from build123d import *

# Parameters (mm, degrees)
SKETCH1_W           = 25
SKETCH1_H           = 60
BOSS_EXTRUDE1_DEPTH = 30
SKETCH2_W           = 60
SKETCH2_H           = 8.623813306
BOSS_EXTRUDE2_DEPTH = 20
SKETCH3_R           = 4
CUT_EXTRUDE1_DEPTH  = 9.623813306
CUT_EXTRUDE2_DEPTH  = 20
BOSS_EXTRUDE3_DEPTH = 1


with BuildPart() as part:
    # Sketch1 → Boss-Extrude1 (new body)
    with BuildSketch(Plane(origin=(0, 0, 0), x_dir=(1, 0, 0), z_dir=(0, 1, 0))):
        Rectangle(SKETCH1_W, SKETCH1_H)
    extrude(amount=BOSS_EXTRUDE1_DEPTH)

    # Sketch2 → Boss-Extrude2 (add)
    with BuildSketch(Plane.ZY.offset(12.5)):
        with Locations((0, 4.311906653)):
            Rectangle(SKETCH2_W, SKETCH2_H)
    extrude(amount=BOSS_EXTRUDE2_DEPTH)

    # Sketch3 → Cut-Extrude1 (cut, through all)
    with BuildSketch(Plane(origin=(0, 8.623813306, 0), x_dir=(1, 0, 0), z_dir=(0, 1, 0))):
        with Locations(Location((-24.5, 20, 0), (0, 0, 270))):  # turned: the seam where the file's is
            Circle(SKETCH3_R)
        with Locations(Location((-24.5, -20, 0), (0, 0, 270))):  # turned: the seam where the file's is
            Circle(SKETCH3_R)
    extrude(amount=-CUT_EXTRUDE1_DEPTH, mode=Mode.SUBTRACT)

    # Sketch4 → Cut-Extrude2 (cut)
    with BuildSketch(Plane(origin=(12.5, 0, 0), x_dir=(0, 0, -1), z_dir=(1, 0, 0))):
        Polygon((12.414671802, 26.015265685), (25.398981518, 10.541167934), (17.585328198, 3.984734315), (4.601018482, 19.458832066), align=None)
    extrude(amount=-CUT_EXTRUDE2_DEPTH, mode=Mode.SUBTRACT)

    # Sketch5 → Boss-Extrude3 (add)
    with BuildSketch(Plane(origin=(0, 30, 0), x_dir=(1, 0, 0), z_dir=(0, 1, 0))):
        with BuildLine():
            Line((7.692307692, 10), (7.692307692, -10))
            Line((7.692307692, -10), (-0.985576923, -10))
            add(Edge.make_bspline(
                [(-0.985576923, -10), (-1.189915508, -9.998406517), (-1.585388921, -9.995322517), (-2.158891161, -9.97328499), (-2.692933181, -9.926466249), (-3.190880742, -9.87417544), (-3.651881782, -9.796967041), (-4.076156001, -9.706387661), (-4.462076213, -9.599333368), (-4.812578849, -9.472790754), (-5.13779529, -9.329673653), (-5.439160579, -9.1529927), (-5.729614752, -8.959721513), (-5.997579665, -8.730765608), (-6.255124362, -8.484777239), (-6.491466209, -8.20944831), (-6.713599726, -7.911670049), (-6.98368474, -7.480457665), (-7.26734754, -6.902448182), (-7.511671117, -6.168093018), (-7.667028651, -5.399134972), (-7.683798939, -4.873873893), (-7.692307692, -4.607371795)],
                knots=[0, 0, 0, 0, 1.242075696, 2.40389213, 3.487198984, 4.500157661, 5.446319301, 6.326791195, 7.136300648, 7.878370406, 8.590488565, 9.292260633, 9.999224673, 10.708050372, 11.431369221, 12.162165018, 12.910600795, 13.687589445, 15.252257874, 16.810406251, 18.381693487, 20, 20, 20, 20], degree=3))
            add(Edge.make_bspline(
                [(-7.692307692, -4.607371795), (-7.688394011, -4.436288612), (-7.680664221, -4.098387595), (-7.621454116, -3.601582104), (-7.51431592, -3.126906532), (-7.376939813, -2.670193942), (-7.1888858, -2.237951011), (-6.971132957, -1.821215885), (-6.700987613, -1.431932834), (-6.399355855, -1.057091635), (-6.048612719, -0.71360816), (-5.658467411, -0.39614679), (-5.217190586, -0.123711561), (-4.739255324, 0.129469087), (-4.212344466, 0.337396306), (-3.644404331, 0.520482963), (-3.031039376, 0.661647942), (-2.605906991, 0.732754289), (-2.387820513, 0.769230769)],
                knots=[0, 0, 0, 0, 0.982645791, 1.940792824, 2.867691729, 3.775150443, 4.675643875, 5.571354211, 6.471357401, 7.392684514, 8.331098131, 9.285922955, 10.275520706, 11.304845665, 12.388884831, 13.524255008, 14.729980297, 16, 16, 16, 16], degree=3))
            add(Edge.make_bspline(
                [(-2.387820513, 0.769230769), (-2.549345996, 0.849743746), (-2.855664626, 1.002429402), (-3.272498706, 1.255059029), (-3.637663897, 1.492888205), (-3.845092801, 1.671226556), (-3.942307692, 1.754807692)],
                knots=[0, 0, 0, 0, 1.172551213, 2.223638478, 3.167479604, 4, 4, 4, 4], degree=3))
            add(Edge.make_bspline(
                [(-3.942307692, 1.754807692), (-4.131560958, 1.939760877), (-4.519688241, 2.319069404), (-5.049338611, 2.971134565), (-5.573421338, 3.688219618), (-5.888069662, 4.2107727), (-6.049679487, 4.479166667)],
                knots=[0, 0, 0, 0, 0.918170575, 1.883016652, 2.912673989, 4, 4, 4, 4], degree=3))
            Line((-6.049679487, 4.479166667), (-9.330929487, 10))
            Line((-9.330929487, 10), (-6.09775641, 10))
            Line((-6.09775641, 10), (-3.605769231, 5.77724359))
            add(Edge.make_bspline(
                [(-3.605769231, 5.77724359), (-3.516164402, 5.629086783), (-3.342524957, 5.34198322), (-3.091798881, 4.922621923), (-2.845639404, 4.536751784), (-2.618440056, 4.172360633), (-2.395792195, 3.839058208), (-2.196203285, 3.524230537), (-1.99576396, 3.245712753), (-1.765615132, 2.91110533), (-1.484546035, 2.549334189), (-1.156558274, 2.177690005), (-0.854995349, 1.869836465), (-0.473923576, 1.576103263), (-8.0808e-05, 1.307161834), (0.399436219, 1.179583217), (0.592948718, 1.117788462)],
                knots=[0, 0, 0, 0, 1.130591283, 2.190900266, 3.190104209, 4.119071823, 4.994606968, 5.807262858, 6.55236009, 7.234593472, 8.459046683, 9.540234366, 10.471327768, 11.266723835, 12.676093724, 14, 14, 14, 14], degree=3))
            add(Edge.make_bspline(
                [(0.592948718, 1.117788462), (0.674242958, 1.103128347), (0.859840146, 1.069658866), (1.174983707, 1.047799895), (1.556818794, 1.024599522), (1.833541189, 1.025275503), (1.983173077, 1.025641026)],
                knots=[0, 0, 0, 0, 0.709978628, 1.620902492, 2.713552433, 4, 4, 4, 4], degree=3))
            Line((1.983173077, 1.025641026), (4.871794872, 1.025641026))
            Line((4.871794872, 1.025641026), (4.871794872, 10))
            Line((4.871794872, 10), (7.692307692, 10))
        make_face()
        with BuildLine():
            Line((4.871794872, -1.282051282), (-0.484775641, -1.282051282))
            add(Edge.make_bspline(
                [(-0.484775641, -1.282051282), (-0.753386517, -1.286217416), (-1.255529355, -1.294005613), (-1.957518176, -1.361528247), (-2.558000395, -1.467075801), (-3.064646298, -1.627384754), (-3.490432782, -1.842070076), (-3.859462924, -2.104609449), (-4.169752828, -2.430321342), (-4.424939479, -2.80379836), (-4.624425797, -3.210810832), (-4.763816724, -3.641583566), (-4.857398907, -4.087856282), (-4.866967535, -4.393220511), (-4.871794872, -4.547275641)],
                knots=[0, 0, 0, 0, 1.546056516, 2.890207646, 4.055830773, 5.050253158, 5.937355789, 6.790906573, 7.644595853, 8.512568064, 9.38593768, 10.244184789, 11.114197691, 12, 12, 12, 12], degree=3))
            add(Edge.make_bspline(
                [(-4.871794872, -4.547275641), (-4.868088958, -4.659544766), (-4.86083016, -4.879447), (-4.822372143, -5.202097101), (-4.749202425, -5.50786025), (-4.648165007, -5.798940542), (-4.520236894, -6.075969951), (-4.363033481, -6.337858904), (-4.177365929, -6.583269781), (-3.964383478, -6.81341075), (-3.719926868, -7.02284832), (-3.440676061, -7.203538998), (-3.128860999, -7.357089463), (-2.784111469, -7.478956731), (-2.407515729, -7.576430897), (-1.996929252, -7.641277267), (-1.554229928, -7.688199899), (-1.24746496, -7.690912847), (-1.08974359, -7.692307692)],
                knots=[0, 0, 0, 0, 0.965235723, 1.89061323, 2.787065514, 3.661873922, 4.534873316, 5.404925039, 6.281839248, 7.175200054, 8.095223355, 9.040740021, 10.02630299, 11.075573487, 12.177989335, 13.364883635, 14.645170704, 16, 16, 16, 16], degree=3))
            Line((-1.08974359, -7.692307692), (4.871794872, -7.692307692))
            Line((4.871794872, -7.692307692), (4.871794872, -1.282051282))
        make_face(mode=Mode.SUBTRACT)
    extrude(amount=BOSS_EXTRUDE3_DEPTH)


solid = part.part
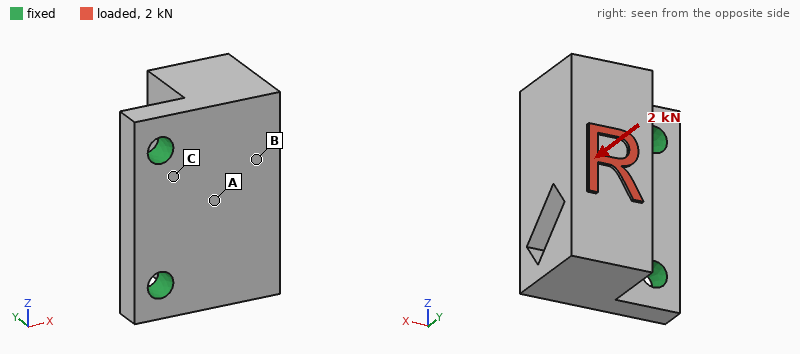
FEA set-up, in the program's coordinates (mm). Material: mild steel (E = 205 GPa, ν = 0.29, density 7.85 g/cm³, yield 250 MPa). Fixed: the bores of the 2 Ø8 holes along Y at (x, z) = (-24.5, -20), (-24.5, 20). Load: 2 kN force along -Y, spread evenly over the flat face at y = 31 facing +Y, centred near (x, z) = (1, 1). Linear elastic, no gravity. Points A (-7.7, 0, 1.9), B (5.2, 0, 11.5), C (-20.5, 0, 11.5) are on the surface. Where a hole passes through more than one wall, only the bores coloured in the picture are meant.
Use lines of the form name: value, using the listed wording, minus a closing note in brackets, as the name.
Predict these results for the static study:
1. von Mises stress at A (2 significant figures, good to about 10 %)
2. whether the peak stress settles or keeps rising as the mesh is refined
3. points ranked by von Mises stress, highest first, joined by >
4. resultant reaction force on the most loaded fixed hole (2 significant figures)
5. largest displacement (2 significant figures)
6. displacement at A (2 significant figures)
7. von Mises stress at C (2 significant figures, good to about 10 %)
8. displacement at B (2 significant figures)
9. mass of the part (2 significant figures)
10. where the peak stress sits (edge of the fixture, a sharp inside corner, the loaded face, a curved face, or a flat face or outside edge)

von Mises stress at A: 16 MPa
whether the peak stress settles or keeps rising as the mesh is refined: keeps rising
points ranked by von Mises stress, highest first, joined by >: C > A > B
resultant reaction force on the most loaded fixed hole: 1.0 kN
largest displacement: 34 µm
displacement at A: 9.8 µm
von Mises stress at C: 34 MPa
displacement at B: 20 µm
mass of the part: 400 g
where the peak stress sits: edge of the fixture
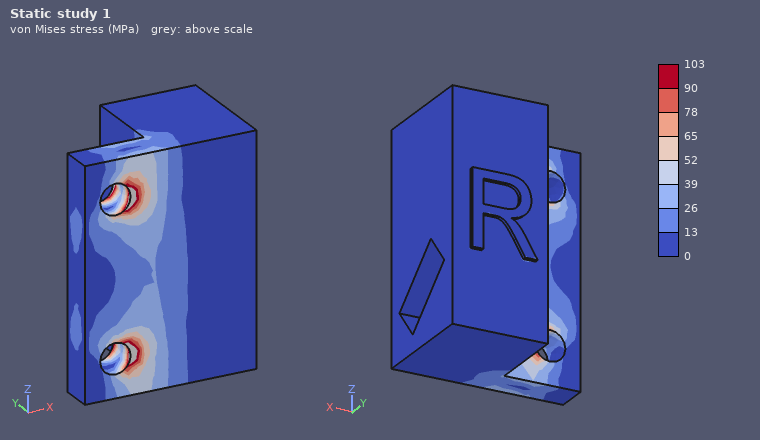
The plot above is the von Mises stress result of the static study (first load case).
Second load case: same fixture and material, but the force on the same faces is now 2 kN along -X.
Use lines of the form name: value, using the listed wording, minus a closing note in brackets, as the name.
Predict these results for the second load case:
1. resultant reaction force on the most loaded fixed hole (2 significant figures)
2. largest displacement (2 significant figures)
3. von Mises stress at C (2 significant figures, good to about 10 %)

resultant reaction force on the most loaded fixed hole: 1.1 kN
largest displacement: 52 µm
von Mises stress at C: 43 MPa
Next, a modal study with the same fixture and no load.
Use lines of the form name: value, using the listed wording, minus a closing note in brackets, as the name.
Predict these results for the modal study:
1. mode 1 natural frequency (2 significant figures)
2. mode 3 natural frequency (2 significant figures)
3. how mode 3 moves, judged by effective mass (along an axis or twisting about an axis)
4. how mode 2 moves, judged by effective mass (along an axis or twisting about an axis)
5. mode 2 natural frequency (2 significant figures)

mode 1 natural frequency: 2500 Hz
mode 3 natural frequency: 10 kHz
how mode 3 moves, judged by effective mass: along Z
how mode 2 moves, judged by effective mass: along Z
mode 2 natural frequency: 6900 Hz
